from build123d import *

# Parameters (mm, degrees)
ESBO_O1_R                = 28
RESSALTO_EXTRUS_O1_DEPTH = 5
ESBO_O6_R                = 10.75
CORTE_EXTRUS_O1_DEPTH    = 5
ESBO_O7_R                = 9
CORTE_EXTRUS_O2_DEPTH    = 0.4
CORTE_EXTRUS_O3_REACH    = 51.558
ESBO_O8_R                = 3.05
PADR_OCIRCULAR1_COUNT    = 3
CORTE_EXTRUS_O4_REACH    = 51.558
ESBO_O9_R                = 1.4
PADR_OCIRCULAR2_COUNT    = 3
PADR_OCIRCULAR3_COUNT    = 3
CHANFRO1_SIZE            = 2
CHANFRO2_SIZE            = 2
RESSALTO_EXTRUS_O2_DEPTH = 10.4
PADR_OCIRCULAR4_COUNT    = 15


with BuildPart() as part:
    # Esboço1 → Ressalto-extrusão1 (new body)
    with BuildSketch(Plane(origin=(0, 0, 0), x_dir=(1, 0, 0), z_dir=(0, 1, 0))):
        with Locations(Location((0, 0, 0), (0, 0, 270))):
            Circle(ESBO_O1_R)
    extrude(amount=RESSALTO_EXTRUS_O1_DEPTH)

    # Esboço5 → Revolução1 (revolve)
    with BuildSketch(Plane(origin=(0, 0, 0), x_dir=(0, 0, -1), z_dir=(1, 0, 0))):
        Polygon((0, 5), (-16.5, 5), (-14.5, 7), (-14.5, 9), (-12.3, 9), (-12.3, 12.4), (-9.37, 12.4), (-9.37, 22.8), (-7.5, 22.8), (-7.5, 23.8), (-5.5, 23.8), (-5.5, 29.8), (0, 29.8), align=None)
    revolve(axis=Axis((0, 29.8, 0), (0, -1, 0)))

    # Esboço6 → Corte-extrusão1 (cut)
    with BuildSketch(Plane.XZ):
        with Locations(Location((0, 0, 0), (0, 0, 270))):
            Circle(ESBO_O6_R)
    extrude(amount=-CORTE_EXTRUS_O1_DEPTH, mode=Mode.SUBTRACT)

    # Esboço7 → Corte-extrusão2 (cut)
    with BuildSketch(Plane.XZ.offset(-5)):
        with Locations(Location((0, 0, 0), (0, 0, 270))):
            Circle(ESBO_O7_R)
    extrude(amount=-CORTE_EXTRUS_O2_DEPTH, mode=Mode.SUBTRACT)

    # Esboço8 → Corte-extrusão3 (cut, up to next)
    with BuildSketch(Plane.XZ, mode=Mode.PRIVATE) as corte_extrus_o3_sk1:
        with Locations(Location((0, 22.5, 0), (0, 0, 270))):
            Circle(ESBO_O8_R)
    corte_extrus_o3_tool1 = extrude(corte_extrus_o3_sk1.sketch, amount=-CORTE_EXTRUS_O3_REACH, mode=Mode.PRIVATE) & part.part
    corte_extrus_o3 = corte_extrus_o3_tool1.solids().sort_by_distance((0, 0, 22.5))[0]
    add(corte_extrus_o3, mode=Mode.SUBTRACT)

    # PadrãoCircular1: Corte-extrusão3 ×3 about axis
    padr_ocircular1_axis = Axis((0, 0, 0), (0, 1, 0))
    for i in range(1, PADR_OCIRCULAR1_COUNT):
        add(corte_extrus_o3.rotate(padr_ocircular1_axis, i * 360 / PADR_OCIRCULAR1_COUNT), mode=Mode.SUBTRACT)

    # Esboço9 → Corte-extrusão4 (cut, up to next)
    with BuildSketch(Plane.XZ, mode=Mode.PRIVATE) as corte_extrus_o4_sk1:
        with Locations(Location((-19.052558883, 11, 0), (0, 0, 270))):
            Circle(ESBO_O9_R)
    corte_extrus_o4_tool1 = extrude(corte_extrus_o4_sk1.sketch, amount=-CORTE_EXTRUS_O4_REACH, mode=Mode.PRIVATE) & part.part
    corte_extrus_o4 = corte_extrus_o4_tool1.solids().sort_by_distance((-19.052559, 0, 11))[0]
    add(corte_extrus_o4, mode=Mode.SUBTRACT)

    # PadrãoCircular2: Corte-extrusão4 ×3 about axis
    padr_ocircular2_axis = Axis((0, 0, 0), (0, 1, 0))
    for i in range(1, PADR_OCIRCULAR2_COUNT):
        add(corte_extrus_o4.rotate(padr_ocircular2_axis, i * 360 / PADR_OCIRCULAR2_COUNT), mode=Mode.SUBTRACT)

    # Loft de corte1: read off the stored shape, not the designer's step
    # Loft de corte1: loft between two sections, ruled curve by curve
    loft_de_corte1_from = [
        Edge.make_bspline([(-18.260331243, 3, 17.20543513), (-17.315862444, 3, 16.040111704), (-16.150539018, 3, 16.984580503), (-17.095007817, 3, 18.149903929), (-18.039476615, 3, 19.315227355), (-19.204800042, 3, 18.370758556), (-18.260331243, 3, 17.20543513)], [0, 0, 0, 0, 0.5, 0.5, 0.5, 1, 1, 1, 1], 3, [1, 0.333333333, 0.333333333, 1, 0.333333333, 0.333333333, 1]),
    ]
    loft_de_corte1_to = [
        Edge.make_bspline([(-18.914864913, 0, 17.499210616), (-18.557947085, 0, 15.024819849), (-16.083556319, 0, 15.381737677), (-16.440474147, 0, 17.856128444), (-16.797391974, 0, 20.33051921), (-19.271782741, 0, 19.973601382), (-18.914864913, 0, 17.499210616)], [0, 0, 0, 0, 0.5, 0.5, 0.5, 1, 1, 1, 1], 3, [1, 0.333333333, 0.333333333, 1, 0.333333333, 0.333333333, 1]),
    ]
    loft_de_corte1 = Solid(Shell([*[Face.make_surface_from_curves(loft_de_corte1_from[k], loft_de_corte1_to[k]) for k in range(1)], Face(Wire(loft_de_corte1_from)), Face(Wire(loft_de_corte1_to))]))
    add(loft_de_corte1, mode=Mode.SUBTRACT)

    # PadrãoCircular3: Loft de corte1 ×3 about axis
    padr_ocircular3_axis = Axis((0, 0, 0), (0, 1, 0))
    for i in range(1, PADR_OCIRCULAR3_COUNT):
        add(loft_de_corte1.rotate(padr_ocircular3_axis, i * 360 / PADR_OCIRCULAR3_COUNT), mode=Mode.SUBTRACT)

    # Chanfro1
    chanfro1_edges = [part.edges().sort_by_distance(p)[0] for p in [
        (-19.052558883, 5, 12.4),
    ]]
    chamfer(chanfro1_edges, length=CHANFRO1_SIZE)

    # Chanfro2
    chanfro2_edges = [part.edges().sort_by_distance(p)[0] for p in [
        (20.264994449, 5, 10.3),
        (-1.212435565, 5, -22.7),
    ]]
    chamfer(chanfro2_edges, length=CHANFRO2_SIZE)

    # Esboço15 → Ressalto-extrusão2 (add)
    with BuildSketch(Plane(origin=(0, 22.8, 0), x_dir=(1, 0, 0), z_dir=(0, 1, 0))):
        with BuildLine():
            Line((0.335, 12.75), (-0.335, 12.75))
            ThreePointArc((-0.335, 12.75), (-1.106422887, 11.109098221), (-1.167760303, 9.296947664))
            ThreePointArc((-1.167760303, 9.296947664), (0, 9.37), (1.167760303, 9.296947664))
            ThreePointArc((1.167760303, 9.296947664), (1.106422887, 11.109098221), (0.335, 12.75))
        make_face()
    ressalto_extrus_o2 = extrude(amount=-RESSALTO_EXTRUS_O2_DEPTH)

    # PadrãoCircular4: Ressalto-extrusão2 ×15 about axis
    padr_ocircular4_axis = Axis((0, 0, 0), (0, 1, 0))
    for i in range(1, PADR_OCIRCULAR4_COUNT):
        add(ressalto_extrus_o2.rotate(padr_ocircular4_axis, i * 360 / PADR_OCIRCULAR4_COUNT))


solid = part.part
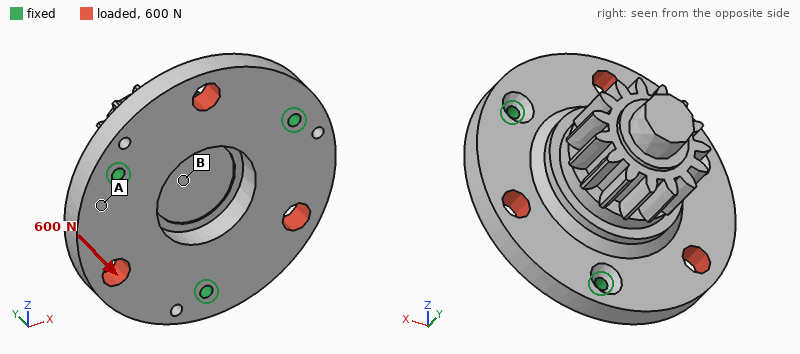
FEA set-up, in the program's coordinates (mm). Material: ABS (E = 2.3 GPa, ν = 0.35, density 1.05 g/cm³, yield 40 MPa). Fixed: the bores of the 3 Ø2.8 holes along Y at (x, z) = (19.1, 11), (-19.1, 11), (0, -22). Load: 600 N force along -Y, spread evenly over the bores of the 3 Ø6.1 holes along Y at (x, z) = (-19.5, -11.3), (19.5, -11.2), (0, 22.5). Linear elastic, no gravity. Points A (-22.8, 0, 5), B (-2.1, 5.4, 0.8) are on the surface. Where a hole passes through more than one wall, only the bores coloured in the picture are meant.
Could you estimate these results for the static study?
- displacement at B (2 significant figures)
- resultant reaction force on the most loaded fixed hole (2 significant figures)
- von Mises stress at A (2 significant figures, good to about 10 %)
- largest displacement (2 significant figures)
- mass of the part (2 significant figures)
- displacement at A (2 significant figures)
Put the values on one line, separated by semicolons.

0.091 mm; 250 N; 6.3 MPa; 0.38 mm; 20 g; 0.063 mm
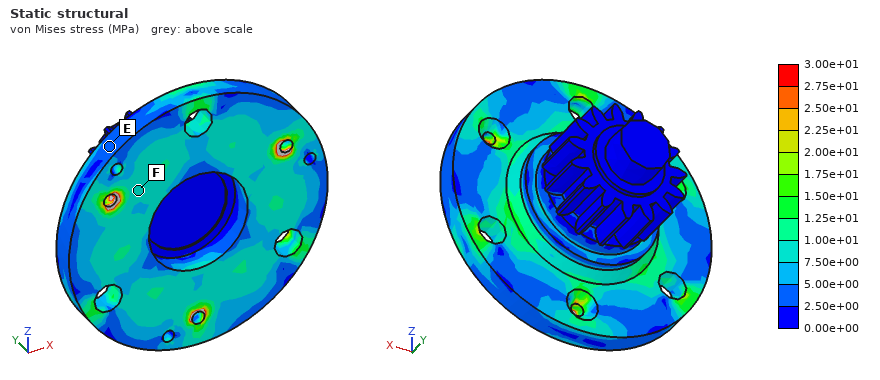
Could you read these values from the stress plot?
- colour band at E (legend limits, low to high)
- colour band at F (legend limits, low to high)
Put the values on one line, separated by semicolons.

2.50e+00 to 5.00e+00 MPa; 7.50e+00 to 1.00e+01 MPa
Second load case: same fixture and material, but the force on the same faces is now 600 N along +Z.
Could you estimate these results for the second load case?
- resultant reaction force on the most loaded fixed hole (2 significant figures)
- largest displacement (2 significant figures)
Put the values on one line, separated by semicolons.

230 N; 54 µm
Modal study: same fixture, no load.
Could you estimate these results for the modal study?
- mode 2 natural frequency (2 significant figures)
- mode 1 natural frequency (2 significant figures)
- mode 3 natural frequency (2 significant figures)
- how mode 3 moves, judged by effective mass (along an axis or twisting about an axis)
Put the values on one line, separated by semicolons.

2800 Hz; 2800 Hz; 3100 Hz; along Y
